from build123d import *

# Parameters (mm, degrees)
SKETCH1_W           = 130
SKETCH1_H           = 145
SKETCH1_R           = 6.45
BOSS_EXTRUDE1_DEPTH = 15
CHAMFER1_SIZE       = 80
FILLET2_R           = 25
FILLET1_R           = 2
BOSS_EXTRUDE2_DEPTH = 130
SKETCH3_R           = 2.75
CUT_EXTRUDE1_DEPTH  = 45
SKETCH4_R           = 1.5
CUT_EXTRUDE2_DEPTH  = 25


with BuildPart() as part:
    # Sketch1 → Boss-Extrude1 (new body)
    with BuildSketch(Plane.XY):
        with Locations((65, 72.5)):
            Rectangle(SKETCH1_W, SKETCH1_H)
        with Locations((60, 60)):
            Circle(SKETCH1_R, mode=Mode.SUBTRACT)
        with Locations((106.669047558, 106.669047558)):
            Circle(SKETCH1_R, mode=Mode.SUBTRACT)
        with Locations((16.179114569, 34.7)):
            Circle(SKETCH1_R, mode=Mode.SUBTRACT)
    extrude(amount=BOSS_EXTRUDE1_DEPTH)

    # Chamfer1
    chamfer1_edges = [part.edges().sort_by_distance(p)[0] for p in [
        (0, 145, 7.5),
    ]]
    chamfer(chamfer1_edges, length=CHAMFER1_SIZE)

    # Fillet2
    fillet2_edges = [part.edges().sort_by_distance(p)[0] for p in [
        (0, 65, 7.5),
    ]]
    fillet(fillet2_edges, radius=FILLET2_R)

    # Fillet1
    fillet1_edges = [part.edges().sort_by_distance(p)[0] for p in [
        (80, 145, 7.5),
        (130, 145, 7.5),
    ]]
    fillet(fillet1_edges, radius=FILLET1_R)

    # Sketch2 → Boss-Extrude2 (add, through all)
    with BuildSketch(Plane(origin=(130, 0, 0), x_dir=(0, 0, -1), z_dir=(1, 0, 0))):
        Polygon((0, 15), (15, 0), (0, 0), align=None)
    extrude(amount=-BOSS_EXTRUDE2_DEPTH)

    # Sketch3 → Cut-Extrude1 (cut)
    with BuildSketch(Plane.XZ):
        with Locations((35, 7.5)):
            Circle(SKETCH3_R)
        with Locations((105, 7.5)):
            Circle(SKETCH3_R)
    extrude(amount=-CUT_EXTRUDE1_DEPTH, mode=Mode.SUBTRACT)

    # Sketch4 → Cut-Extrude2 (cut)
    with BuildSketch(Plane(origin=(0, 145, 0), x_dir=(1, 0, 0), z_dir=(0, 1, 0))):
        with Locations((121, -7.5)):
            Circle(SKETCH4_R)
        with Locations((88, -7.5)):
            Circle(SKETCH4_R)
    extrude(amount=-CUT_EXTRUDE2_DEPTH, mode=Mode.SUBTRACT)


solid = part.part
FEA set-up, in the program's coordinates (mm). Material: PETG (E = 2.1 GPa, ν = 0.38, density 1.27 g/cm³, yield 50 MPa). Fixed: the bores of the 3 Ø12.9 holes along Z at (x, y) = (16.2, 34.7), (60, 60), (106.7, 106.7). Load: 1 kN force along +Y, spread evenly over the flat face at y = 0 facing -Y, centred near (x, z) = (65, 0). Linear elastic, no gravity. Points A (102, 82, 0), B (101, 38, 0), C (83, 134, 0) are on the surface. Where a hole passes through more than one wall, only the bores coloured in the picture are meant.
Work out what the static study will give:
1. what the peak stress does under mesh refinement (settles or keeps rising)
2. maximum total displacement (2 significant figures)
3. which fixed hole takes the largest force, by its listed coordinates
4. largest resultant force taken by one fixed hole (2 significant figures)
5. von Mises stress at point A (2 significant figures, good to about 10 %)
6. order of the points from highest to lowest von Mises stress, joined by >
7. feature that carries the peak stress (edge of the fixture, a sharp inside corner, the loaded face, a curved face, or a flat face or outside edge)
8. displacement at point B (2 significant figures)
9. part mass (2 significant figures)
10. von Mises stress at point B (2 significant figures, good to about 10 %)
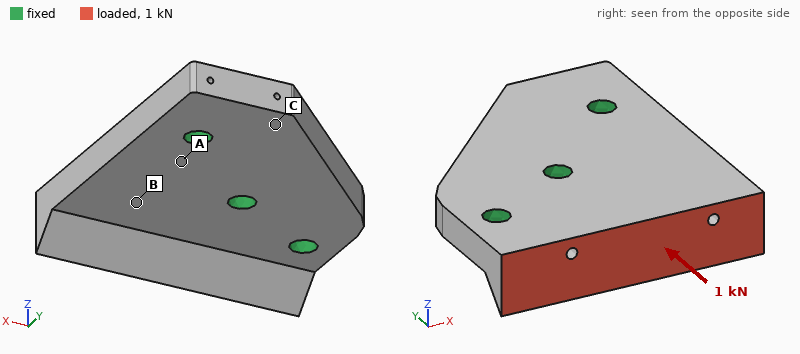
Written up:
keeps rising
0.24 mm
(60, 60)
410 N
0.79 MPa
B > A > C
edge of the fixture
0.048 mm
310 g
1.5 MPa
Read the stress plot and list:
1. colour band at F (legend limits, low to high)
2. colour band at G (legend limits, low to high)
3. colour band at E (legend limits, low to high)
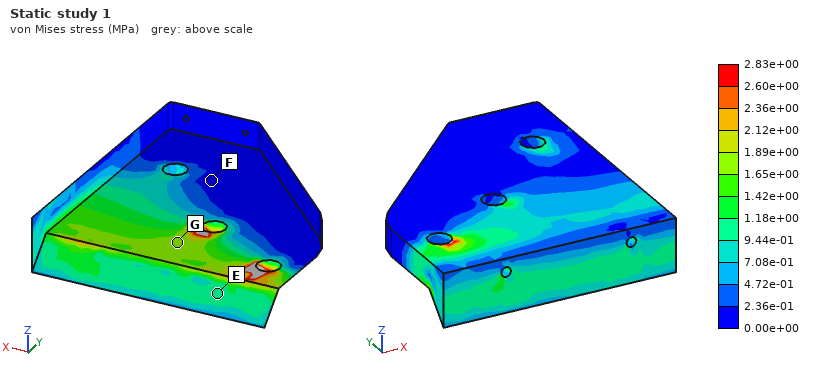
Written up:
0.00e+00 to 2.36e-01 MPa
1.65e+00 to 1.89e+00 MPa
9.44e-01 to 1.18e+00 MPa
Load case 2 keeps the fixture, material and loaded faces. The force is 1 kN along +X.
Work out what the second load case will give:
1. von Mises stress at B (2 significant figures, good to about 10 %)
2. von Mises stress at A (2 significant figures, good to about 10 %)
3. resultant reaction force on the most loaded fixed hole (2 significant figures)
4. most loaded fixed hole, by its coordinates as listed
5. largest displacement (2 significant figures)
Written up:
0.92 MPa
0.44 MPa
800 N
(16.2, 34.7)
0.21 mm
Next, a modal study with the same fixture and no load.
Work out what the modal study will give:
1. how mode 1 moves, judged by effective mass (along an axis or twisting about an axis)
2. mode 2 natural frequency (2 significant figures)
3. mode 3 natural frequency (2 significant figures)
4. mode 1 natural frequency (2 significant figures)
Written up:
along Z
1500 Hz
1500 Hz
590 Hz
